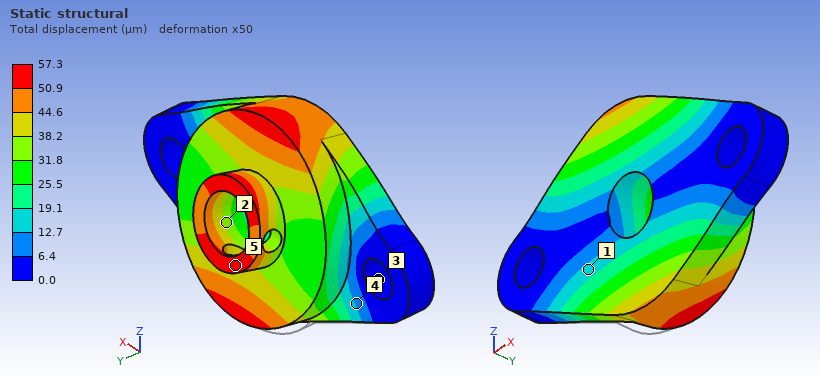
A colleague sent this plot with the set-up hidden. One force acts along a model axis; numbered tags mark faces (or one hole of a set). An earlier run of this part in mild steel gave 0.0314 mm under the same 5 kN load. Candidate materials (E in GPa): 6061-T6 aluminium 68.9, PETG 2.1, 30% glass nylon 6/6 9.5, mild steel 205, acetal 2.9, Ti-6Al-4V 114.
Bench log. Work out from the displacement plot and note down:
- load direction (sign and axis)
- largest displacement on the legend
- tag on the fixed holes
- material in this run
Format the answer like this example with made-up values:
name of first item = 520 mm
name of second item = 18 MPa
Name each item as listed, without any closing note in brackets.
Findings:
load direction = +Z
largest displacement on the legend = 57.3 µm
tag on the fixed holes = 3
material in this run = Ti-6Al-4V
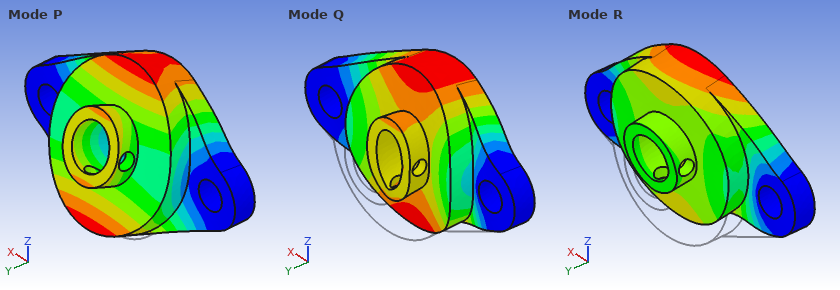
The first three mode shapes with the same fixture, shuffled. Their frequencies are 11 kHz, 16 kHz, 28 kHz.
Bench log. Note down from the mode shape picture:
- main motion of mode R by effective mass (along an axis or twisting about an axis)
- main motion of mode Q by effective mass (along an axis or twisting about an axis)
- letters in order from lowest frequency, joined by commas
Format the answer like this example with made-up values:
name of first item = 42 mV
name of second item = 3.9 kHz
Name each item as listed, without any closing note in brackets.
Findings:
main motion of mode R by effective mass = along Z
main motion of mode Q by effective mass = along Y
letters in order from lowest frequency, joined by commas = P, Q, R
